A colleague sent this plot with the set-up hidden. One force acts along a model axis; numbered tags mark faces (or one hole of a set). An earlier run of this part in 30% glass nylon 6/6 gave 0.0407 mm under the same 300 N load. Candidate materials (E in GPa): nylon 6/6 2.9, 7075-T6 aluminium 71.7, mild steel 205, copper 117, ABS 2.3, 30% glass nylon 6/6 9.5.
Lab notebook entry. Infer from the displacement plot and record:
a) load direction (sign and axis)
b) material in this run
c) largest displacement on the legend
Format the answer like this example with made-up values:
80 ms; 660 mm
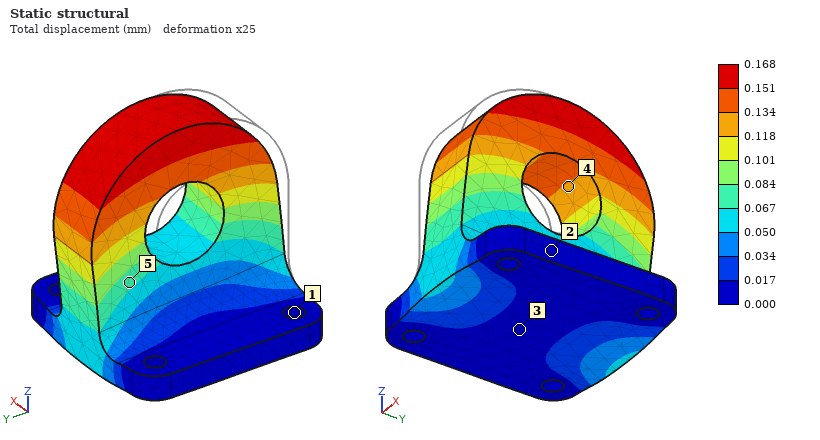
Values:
+Y; ABS; 0.168 mm
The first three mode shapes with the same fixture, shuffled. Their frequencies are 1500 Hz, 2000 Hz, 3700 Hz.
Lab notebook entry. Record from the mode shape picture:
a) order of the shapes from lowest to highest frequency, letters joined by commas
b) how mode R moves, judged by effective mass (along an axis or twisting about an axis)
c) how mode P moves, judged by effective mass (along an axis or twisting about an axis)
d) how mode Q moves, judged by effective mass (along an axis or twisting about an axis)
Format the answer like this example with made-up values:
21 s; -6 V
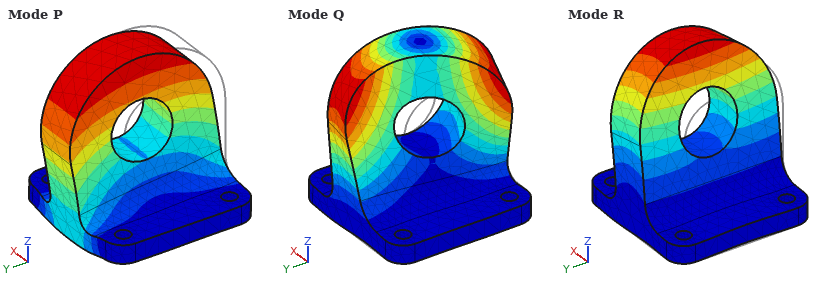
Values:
R, P, Q; along X; along Y; twisting about Z
